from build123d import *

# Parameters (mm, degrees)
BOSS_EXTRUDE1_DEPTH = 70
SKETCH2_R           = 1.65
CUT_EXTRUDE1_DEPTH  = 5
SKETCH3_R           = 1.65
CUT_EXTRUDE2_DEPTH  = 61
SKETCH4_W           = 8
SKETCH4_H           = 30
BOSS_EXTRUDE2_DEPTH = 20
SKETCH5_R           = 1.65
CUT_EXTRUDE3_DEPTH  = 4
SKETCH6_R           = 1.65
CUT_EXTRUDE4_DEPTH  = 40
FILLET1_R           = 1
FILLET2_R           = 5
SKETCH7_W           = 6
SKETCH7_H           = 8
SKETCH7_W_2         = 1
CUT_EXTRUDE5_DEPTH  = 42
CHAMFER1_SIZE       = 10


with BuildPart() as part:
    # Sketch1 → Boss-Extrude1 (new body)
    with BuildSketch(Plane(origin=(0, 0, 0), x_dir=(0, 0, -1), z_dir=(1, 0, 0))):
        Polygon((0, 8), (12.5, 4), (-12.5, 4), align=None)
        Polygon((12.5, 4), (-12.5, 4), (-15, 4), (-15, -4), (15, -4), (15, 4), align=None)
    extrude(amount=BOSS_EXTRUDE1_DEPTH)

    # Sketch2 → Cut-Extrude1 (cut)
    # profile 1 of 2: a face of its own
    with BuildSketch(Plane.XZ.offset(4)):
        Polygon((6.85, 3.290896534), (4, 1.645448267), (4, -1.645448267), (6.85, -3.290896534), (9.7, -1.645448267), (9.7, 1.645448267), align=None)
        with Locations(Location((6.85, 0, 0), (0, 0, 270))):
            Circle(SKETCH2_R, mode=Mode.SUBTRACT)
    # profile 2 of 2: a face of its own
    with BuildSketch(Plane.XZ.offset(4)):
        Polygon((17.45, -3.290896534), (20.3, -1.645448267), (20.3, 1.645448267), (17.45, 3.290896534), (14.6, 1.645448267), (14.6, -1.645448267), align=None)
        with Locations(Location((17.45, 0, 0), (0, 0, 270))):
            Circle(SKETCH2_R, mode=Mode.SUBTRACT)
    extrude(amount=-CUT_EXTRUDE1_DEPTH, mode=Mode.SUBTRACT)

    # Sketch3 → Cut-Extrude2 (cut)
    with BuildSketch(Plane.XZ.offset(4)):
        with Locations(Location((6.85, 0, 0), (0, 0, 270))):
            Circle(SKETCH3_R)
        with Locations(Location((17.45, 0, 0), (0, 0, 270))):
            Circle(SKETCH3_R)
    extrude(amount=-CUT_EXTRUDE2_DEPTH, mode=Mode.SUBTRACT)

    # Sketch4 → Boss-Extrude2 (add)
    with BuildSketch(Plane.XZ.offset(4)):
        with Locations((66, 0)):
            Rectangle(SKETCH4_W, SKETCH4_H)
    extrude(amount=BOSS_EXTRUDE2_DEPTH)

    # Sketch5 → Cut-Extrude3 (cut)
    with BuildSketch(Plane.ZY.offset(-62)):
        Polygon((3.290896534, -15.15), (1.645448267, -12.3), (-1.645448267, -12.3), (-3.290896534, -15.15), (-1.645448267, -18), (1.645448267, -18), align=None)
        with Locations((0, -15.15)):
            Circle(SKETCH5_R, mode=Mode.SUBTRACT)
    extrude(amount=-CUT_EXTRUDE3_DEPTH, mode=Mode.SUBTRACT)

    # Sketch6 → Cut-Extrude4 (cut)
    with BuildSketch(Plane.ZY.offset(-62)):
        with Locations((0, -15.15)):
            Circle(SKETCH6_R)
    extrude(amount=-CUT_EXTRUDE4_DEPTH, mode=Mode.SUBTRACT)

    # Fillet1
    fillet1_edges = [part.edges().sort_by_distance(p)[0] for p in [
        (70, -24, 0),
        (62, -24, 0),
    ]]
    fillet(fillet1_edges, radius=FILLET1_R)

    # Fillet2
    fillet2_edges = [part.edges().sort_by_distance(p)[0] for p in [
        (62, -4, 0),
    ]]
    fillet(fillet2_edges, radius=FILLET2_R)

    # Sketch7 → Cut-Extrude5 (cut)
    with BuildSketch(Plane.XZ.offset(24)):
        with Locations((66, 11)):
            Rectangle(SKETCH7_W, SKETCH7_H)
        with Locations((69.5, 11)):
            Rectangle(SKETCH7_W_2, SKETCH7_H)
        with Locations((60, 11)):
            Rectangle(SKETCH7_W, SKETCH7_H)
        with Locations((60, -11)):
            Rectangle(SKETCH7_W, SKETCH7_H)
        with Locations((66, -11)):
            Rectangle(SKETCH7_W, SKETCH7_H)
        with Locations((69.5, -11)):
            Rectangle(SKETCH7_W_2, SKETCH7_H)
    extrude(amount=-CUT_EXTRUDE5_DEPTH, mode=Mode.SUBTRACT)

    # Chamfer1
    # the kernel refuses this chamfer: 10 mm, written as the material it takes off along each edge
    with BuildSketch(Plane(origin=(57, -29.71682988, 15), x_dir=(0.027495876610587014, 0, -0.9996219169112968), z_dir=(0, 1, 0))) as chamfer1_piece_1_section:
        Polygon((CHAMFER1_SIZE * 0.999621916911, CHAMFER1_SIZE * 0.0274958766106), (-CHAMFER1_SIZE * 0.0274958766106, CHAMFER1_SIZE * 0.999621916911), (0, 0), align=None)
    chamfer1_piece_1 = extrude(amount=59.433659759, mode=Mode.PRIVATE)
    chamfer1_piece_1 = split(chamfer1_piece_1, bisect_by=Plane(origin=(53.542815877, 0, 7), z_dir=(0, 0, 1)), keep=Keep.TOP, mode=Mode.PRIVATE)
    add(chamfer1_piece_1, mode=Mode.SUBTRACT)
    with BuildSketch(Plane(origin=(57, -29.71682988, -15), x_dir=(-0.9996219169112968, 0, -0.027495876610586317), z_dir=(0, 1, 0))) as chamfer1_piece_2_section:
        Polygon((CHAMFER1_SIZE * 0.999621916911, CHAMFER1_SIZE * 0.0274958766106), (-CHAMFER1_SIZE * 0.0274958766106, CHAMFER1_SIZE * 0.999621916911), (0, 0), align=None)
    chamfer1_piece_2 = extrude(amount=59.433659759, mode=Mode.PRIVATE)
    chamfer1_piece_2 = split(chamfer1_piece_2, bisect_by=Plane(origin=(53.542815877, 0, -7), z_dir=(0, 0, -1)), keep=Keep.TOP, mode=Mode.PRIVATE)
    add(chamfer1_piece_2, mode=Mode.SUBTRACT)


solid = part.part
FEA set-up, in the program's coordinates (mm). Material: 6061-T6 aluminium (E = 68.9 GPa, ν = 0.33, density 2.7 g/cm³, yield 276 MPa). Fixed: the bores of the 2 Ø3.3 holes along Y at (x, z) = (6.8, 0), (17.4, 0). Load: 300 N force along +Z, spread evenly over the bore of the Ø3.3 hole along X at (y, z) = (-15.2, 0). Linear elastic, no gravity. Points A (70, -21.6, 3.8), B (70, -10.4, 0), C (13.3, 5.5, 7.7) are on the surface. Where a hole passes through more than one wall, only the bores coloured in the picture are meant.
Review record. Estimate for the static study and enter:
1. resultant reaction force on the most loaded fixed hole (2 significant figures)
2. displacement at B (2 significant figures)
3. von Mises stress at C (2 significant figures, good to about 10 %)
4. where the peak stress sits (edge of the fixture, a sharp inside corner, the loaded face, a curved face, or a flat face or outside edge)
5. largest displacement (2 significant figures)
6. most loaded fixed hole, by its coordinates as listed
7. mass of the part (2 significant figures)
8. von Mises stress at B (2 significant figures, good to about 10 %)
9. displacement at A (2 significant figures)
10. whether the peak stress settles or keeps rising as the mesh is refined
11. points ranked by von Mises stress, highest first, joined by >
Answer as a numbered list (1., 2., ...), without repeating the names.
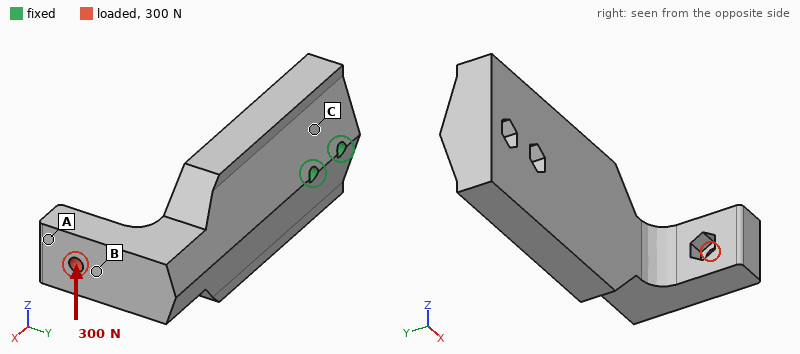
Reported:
1. 1.4 kN
2. 62 µm
3. 21 MPa
4. edge of the fixture
5. 92 µm
6. (17.4, 0)
7. 53 g
8. 10 MPa
9. 87 µm
10. keeps rising
11. C > B > A
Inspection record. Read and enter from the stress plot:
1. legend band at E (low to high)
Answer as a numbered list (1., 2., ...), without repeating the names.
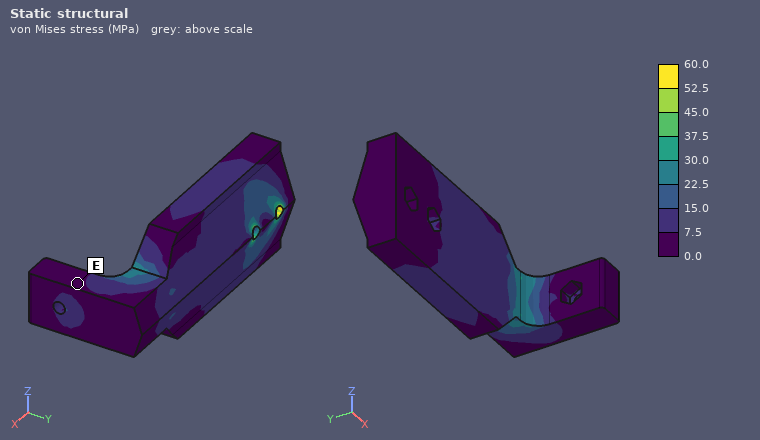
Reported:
1. 0.0 to 7.5 MPa
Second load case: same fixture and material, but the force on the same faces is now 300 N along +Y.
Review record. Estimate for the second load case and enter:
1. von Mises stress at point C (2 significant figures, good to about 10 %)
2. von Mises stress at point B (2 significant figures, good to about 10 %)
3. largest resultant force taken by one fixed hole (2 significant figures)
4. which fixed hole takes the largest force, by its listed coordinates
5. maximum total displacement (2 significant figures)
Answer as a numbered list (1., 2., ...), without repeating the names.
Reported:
1. 11 MPa
2. 8.1 MPa
3. 1.2 kN
4. (17.4, 0)
5. 0.14 mm
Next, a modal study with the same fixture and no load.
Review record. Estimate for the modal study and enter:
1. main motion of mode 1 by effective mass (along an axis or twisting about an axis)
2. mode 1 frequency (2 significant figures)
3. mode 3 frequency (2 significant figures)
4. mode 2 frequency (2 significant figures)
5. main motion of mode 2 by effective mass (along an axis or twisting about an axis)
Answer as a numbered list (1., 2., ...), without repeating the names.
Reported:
1. along Y
2. 2300 Hz
3. 6900 Hz
4. 3500 Hz
5. along Z
